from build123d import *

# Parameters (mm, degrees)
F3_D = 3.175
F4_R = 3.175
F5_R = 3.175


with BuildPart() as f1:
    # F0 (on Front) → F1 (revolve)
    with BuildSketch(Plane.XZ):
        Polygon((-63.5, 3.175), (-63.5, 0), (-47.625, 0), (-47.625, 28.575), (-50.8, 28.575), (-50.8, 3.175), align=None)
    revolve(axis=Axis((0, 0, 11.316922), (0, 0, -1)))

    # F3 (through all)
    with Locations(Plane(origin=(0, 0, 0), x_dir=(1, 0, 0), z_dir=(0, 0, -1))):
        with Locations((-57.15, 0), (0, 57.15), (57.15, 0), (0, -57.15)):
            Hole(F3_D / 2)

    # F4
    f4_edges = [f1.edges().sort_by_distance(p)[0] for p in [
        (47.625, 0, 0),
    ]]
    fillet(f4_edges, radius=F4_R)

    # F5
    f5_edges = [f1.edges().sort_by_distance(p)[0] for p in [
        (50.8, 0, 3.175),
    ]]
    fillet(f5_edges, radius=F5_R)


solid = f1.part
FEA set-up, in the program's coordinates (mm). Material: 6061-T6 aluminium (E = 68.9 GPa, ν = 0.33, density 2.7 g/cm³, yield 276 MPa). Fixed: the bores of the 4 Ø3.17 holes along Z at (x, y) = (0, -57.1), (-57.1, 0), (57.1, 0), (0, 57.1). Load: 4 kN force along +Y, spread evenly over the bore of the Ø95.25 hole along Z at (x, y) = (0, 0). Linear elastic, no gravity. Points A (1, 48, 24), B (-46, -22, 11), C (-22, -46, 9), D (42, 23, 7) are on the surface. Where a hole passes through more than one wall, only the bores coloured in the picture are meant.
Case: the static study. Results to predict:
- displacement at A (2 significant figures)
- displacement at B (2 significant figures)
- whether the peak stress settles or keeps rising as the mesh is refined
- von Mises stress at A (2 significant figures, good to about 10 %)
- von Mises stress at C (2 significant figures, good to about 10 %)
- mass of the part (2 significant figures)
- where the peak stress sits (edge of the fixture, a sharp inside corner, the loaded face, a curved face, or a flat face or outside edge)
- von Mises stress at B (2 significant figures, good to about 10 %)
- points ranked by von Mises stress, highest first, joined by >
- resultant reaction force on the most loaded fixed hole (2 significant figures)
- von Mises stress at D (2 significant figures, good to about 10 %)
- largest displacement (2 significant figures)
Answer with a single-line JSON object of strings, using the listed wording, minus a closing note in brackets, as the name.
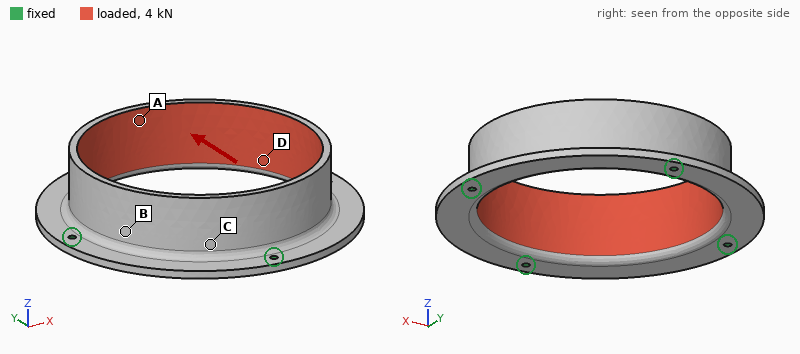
{"displacement at A": "14 µm", "displacement at B": "26 µm", "whether the peak stress settles or keeps rising as the mesh is refined": "keeps rising", "von Mises stress at A": "27 MPa", "von Mises stress at C": "17 MPa", "mass of the part": "110 g", "where the peak stress sits": "edge of the fixture", "von Mises stress at B": "5.4 MPa", "points ranked by von Mises stress, highest first, joined by >": "A > C > D > B", "resultant reaction force on the most loaded fixed hole": "1.4 kN", "von Mises stress at D": "11 MPa", "largest displacement": "54 µm"}
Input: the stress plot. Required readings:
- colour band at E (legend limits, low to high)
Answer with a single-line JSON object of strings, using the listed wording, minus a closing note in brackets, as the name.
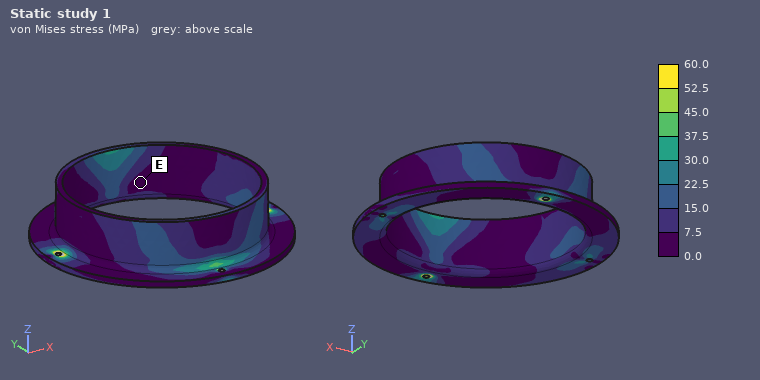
{"colour band at E": "0.0 to 7.5 MPa"}
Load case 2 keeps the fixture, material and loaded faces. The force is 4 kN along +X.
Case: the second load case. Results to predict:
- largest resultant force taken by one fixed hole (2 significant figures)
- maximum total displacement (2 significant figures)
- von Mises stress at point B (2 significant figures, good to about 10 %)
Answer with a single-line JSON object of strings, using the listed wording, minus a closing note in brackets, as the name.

{"largest resultant force taken by one fixed hole": "1.4 kN", "maximum total displacement": "53 µm", "von Mises stress at point B": "16 MPa"}
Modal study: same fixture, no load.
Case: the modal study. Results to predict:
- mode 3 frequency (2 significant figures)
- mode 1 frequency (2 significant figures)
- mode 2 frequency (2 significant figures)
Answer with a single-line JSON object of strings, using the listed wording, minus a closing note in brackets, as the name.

{"mode 3 frequency": "3200 Hz", "mode 1 frequency": "2000 Hz", "mode 2 frequency": "3200 Hz"}
